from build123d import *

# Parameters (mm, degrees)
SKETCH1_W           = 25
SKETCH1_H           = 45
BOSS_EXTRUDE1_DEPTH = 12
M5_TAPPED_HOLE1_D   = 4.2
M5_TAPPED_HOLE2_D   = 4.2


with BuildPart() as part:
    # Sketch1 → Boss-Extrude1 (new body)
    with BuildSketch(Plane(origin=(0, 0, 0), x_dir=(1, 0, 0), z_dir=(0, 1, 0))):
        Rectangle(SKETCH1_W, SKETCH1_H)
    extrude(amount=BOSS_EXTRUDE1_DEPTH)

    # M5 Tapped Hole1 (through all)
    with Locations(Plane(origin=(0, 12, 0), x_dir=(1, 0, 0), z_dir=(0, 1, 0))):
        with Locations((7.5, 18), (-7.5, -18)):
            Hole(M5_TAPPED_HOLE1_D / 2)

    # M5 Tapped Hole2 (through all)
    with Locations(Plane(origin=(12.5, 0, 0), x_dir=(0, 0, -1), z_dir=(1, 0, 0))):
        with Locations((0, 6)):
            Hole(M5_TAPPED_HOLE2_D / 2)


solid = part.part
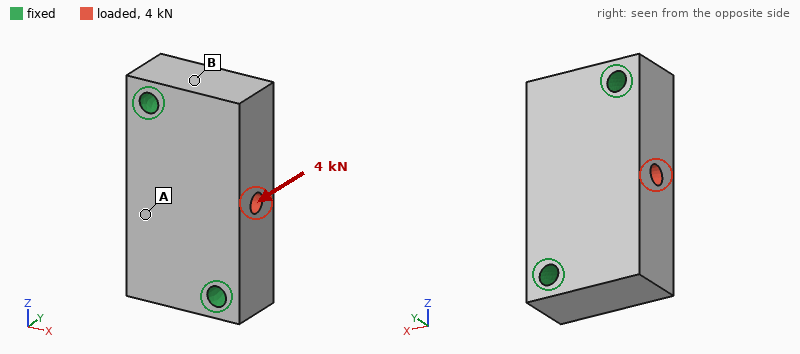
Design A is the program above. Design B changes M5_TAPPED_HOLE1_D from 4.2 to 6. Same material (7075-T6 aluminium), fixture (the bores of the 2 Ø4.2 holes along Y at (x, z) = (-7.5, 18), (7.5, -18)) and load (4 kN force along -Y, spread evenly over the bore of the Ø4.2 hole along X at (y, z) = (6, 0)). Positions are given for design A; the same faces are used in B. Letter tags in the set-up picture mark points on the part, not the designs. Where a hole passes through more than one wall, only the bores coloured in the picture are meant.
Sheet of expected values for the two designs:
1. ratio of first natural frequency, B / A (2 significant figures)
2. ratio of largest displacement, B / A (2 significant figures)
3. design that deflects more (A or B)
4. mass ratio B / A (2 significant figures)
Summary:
1.1
0.86
A
0.97
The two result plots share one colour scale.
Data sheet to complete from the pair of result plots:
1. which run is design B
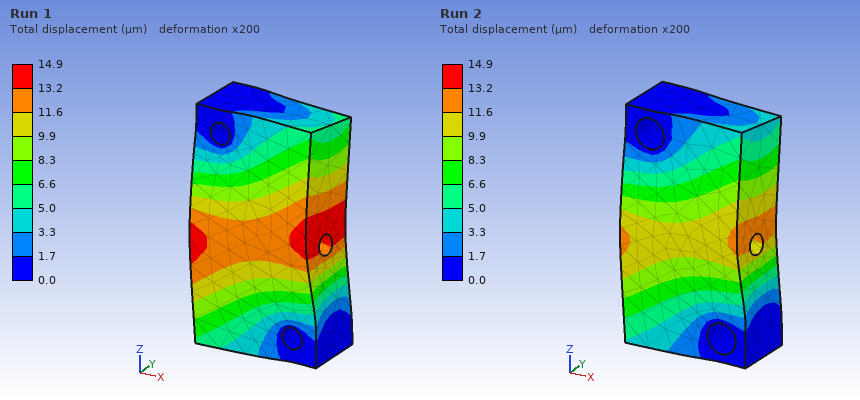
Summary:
Run 2
